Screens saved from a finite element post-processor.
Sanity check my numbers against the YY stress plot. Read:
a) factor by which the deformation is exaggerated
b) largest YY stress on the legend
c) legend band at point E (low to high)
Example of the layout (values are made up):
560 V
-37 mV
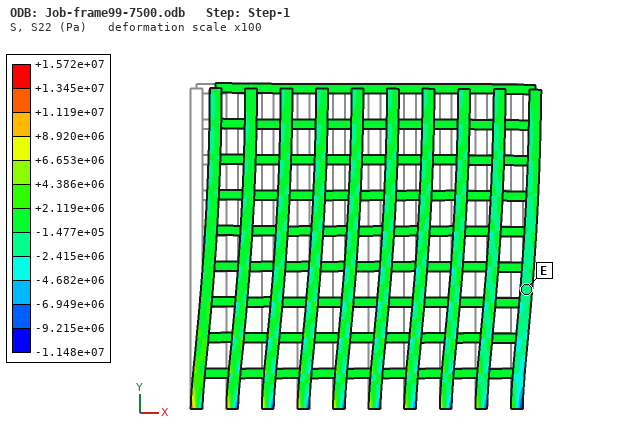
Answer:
100
+1.572e+07 Pa
-2.415e+06 to -1.477e+05 Pa
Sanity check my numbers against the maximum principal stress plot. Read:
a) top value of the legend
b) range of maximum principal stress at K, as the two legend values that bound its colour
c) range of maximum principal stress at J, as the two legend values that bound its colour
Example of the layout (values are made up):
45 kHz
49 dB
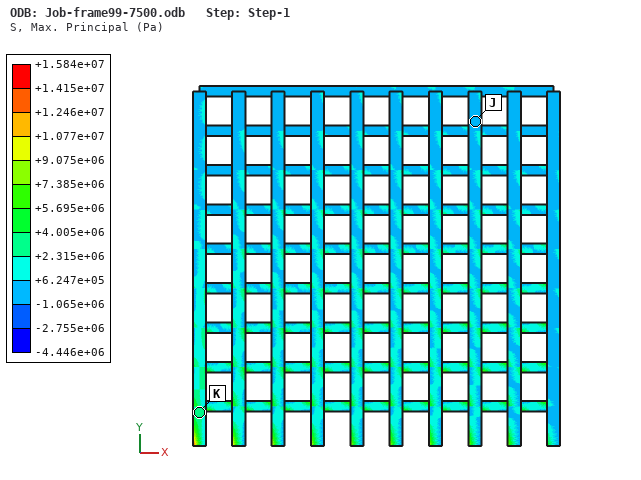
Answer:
+1.584e+07 Pa
+2.315e+06 to +4.005e+06 Pa
-1.065e+06 to +6.247e+05 Pa
